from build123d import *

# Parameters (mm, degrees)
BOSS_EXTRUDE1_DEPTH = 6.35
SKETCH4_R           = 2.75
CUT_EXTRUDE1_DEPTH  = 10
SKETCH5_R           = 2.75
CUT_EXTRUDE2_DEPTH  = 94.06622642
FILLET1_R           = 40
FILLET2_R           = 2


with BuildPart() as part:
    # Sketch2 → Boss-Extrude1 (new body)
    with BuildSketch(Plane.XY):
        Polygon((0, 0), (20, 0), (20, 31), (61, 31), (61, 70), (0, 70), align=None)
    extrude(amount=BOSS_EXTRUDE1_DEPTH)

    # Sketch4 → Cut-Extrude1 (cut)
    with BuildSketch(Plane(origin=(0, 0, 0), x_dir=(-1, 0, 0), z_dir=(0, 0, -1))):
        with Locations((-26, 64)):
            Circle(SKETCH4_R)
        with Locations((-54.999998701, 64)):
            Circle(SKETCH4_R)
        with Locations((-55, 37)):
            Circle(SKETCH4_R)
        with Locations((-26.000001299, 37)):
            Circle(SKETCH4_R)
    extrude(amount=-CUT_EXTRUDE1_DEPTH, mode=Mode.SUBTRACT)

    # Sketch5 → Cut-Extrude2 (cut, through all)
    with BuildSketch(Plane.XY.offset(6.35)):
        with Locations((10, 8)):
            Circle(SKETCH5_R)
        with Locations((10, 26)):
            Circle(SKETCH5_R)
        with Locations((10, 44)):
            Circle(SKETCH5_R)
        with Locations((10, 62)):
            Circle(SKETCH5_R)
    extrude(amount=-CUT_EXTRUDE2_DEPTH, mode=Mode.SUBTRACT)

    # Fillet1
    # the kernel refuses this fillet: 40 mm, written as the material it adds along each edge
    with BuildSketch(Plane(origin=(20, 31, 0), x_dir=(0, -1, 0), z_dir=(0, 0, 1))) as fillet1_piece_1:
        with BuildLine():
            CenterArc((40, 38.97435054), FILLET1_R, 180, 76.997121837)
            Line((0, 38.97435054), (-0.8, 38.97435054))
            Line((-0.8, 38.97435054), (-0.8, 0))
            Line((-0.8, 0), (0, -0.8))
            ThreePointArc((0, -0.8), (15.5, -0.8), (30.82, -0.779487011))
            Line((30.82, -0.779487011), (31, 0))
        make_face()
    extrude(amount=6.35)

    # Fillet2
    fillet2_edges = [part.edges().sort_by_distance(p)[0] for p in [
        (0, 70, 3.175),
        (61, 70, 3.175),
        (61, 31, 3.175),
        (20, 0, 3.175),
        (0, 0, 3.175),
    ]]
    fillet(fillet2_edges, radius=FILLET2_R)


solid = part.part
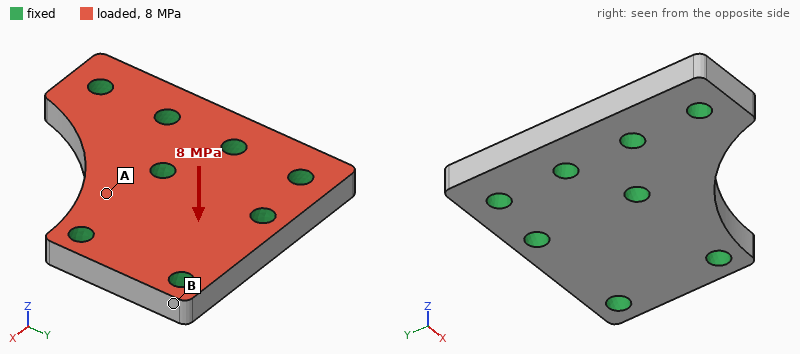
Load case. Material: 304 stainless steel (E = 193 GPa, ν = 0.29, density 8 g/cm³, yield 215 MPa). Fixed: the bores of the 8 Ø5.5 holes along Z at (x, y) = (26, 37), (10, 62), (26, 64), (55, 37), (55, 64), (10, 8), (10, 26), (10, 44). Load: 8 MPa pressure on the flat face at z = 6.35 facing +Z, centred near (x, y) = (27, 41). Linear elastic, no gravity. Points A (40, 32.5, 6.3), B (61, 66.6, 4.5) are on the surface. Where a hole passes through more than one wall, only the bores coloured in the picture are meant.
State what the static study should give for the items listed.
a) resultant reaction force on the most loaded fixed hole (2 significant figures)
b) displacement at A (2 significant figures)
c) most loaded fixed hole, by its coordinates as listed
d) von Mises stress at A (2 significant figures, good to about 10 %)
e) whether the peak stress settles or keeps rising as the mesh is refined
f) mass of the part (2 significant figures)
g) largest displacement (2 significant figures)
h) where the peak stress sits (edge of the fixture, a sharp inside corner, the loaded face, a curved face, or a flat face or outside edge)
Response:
4.7 kN
7.0 µm
(26, 37)
55 MPa
keeps rising
160 g
12 µm
edge of the fixture
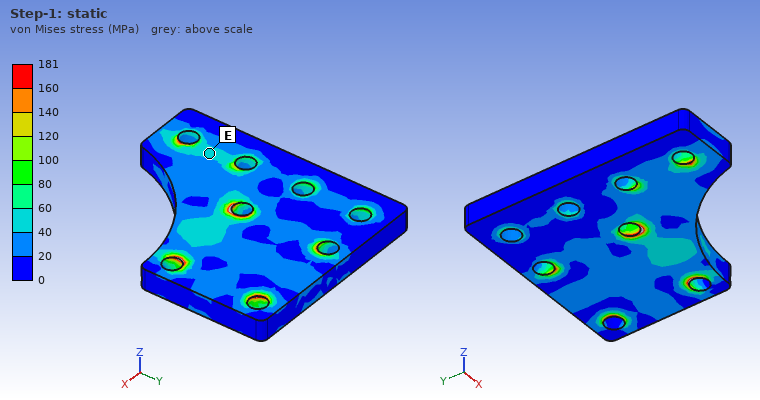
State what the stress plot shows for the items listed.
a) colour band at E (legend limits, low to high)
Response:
40 to 60 MPa
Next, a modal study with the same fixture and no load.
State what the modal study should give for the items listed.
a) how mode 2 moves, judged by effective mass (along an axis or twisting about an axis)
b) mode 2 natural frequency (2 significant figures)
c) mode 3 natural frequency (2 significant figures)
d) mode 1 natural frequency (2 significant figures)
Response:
along Z
28 kHz
35 kHz
23 kHz
